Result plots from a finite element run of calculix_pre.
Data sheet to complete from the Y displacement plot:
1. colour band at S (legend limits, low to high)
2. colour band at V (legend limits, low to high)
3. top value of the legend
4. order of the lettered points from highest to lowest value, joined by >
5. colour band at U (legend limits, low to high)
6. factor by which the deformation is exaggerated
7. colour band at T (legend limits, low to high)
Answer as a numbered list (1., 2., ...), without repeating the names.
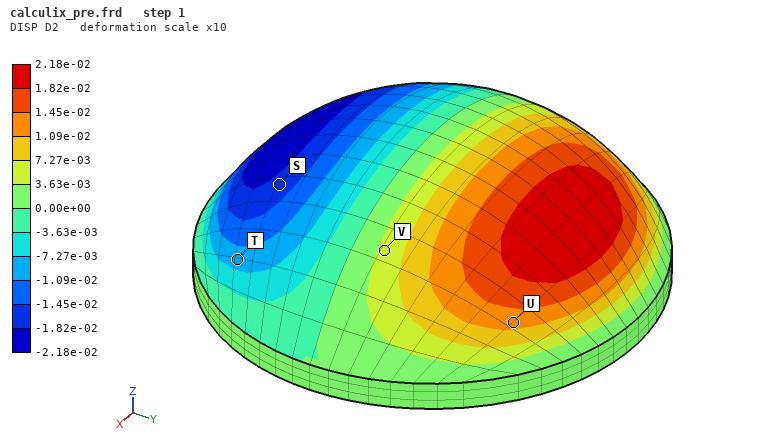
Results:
1. -1.82e-02 to -1.45e-02
2. 3.63e-03 to 7.27e-03
3. 2.18e-02
4. U > V > T > S
5. 1.09e-02 to 1.45e-02
6. 10
7. -1.09e-02 to -7.27e-03
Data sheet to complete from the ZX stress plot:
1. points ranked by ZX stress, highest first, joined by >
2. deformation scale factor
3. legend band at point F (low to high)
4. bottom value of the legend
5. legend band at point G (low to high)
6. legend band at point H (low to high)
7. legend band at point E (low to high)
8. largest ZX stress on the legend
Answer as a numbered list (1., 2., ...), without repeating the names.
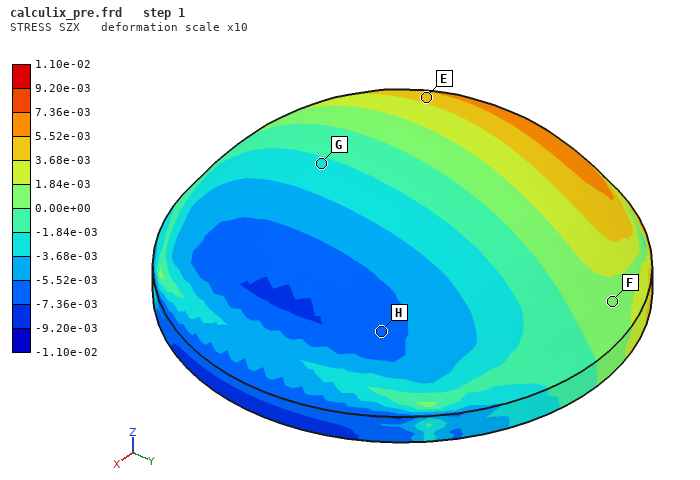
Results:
1. E > F > G > H
2. 10
3. 0.00e+00 to 1.84e-03
4. -1.10e-02
5. -3.68e-03 to -1.84e-03
6. -7.36e-03 to -5.52e-03
7. 3.68e-03 to 5.52e-03
8. 1.10e-02
